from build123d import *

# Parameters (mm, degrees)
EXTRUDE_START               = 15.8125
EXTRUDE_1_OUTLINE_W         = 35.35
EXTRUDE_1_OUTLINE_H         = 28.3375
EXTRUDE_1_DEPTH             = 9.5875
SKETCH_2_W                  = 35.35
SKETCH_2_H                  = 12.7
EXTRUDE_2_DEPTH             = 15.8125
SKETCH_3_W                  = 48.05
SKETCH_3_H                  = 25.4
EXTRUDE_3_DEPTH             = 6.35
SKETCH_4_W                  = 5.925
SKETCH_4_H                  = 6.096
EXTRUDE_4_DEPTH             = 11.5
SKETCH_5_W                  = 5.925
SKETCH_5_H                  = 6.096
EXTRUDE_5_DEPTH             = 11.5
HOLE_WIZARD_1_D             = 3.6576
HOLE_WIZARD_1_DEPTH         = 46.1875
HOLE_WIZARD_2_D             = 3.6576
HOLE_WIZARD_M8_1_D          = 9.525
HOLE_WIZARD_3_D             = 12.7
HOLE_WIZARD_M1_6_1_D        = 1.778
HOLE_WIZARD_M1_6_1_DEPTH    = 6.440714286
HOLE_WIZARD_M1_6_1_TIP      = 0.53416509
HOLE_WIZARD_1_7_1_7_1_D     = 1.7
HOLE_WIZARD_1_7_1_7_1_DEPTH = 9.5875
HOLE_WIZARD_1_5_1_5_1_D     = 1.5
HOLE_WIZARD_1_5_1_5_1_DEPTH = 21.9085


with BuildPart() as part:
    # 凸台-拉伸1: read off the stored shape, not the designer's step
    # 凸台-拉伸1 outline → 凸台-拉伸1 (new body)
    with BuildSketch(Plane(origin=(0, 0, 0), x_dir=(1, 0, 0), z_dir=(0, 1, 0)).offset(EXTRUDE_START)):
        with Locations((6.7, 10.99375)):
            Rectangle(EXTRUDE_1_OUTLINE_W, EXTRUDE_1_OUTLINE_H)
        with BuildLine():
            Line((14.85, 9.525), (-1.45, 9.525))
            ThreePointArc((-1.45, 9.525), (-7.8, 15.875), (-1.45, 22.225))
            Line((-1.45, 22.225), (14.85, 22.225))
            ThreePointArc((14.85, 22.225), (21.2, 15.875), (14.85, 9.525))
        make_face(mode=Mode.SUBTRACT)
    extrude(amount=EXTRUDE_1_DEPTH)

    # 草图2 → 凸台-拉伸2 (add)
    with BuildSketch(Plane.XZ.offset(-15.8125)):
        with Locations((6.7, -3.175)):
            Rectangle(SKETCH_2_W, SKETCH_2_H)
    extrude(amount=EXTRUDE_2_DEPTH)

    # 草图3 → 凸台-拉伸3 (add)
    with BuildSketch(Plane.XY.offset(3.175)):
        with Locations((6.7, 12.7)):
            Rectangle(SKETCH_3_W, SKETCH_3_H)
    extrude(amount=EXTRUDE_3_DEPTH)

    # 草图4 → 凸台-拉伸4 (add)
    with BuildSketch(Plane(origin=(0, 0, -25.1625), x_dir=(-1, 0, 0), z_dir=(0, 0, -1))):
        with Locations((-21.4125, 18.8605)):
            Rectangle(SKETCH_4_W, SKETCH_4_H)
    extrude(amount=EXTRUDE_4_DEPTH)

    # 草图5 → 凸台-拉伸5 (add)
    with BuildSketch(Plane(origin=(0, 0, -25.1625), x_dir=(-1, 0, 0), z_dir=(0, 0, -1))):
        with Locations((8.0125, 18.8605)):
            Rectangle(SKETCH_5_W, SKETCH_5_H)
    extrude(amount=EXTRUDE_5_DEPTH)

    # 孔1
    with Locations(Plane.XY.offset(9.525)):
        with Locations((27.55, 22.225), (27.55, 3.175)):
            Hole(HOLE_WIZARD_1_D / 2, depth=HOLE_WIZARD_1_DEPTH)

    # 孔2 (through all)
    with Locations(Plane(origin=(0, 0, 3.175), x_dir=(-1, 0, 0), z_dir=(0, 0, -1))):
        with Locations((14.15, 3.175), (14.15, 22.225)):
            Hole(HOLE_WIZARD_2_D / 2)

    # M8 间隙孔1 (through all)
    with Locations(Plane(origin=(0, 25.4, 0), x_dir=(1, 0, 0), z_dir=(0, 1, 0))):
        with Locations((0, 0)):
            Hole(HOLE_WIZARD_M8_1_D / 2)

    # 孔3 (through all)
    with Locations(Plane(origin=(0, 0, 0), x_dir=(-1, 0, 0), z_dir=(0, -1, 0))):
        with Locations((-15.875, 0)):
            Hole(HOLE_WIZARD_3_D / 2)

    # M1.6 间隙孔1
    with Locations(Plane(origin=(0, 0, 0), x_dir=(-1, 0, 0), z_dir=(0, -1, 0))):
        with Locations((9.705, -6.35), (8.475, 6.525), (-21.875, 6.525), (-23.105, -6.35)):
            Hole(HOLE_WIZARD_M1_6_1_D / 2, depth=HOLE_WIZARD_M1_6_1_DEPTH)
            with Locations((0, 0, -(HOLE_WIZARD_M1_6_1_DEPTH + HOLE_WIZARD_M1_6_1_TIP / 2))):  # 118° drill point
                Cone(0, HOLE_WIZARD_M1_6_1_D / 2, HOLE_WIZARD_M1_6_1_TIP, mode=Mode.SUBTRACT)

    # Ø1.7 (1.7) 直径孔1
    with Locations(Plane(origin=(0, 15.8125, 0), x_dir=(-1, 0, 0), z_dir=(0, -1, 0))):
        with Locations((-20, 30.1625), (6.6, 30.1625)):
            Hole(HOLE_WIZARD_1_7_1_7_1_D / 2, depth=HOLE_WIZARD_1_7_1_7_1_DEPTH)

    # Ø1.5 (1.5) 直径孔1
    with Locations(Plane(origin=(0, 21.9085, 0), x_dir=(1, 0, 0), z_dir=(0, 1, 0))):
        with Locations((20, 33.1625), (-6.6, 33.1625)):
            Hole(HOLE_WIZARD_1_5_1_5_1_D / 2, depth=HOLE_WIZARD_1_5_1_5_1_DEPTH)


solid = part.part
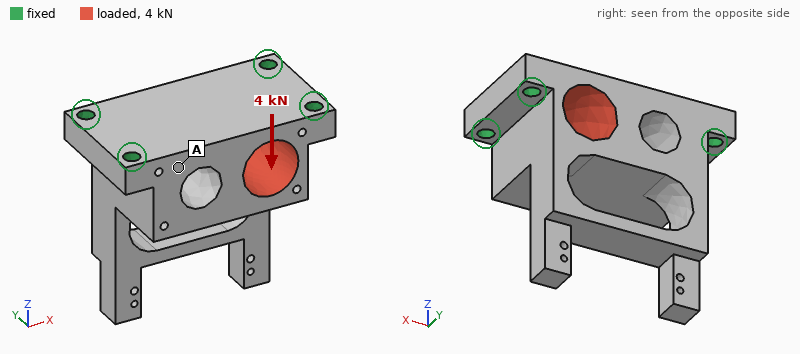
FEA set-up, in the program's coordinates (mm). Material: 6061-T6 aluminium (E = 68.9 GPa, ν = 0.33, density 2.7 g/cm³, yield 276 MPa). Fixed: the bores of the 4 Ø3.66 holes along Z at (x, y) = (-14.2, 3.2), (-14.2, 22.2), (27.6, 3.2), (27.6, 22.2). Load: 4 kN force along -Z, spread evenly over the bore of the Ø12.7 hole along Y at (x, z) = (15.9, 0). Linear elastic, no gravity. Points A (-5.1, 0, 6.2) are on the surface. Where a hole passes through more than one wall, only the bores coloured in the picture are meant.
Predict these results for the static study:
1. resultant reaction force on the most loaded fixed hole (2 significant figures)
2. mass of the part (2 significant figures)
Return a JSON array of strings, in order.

["1.5 kN", "45 g"]
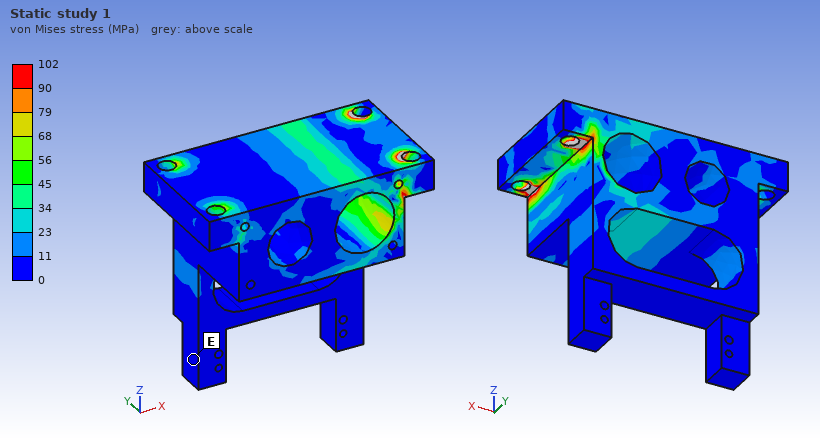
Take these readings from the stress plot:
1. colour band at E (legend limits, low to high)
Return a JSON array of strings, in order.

["0 to 11 MPa"]
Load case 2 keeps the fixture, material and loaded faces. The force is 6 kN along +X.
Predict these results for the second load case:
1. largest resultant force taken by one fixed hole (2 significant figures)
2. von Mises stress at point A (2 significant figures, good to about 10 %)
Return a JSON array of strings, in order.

["1.7 kN", "21 MPa"]
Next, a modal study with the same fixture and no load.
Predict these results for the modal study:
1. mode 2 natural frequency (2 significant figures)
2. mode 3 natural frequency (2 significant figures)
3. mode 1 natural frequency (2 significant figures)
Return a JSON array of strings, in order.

["6000 Hz", "8200 Hz", "6000 Hz"]
